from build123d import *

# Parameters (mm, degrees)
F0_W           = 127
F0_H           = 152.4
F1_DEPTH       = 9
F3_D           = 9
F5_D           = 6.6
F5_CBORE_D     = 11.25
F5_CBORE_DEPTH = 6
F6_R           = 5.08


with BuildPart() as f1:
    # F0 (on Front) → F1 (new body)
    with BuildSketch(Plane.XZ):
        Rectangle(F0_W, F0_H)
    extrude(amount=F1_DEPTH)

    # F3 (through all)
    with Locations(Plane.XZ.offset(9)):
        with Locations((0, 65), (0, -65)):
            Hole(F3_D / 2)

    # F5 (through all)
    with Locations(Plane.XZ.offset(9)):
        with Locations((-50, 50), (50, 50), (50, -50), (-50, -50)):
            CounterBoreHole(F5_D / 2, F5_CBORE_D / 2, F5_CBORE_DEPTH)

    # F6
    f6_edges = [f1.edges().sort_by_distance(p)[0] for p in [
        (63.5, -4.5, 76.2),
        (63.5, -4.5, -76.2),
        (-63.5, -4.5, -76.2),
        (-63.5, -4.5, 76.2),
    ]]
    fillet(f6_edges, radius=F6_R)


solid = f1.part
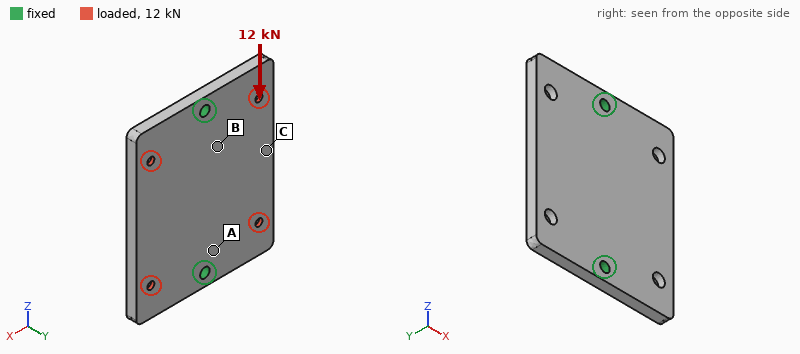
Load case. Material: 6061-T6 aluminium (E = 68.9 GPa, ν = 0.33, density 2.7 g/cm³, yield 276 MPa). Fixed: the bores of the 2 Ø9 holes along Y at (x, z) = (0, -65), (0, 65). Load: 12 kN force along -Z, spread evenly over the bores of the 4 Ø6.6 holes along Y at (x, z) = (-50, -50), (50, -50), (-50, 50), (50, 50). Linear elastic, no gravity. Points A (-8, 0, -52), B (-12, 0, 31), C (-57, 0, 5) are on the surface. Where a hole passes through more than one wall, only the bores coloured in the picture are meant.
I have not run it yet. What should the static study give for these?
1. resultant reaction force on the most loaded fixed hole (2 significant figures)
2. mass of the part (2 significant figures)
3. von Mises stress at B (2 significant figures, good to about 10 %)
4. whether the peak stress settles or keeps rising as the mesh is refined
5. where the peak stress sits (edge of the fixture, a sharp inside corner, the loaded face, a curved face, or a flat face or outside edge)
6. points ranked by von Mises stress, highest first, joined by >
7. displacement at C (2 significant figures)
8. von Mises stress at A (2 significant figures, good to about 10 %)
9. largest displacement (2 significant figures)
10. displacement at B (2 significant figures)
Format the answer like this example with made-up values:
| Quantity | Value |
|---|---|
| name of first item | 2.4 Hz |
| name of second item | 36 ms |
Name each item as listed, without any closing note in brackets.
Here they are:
| Quantity | Value |
|---|---|
| resultant reaction force on the most loaded fixed hole | 6.0 kN |
| mass of the part | 460 g |
| von Mises stress at B | 9.3 MPa |
| whether the peak stress settles or keeps rising as the mesh is refined | keeps rising |
| where the peak stress sits | a sharp inside corner |
| points ranked by von Mises stress, highest first, joined by > | A > B > C |
| displacement at C | 14 µm |
| von Mises stress at A | 19 MPa |
| largest displacement | 39 µm |
| displacement at B | 8.4 µm |
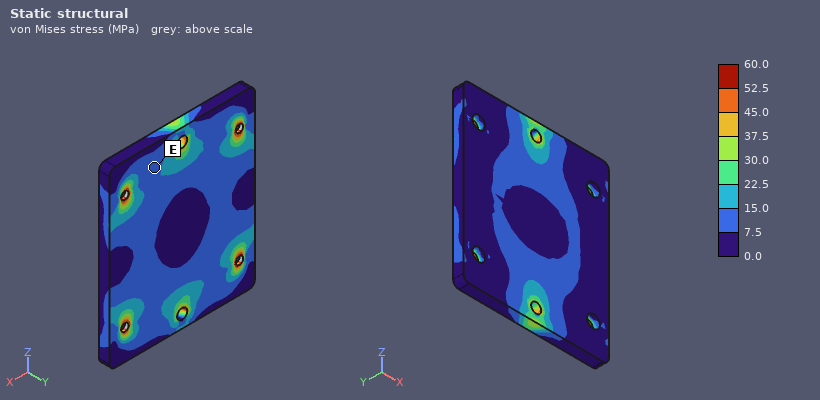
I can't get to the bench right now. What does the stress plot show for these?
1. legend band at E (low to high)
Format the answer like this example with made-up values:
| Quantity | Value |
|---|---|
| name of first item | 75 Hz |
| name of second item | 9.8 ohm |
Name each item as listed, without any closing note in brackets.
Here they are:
| Quantity | Value |
|---|---|
| legend band at E | 7.5 to 15.0 MPa |
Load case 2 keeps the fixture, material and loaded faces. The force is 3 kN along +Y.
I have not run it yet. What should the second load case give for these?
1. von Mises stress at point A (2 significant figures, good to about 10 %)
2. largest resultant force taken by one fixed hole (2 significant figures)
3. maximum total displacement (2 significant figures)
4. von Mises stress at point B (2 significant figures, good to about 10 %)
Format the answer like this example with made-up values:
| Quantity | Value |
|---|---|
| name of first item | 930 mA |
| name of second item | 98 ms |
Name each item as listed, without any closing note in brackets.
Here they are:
| Quantity | Value |
|---|---|
| von Mises stress at point A | 32 MPa |
| largest resultant force taken by one fixed hole | 1.5 kN |
| maximum total displacement | 0.15 mm |
| von Mises stress at point B | 24 MPa |
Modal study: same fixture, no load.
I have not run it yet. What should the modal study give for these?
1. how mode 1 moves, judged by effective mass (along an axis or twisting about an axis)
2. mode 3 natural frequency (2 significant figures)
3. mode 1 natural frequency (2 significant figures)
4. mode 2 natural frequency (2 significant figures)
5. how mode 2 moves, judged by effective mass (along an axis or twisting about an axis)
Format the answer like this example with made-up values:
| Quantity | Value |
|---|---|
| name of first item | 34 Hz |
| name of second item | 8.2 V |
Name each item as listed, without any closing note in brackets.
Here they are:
| Quantity | Value |
|---|---|
| how mode 1 moves, judged by effective mass | twisting about Z |
| mode 3 natural frequency | 2400 Hz |
| mode 1 natural frequency | 1100 Hz |
| mode 2 natural frequency | 1500 Hz |
| how mode 2 moves, judged by effective mass | along Y |
